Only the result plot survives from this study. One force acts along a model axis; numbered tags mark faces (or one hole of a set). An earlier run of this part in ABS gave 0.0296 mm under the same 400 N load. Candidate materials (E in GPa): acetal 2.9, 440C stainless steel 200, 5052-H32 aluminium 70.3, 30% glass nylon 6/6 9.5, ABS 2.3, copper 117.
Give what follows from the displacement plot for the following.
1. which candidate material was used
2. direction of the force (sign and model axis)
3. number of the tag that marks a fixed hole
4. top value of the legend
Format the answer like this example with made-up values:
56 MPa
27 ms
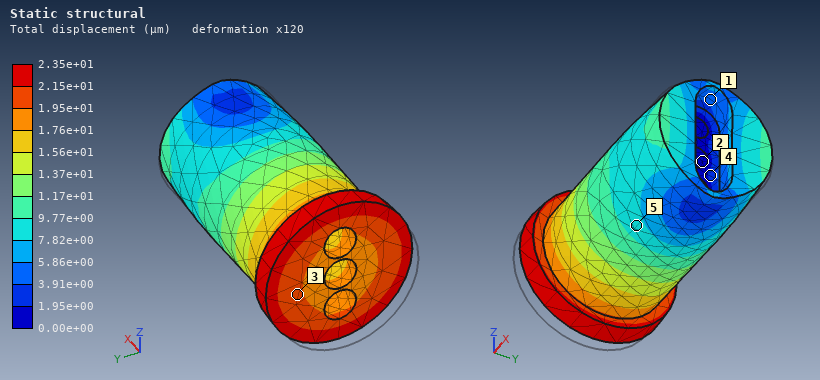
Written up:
acetal
+X
2
2.35e+01 µm
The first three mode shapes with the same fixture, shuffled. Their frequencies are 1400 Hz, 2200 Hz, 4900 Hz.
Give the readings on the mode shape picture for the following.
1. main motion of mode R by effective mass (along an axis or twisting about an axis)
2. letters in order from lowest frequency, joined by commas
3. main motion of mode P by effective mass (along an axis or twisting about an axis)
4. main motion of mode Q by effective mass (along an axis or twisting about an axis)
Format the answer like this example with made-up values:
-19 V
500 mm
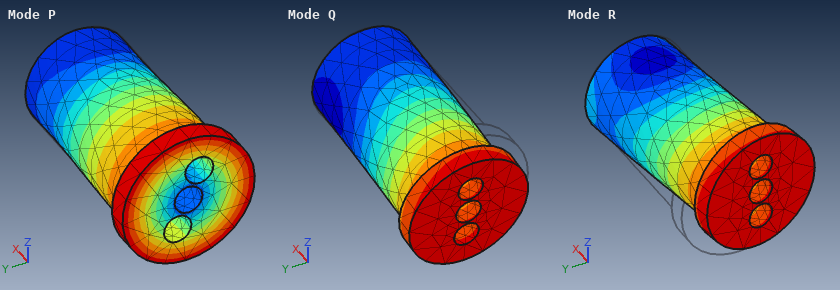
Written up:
along Y
R, Q, P
twisting about X
along Z
